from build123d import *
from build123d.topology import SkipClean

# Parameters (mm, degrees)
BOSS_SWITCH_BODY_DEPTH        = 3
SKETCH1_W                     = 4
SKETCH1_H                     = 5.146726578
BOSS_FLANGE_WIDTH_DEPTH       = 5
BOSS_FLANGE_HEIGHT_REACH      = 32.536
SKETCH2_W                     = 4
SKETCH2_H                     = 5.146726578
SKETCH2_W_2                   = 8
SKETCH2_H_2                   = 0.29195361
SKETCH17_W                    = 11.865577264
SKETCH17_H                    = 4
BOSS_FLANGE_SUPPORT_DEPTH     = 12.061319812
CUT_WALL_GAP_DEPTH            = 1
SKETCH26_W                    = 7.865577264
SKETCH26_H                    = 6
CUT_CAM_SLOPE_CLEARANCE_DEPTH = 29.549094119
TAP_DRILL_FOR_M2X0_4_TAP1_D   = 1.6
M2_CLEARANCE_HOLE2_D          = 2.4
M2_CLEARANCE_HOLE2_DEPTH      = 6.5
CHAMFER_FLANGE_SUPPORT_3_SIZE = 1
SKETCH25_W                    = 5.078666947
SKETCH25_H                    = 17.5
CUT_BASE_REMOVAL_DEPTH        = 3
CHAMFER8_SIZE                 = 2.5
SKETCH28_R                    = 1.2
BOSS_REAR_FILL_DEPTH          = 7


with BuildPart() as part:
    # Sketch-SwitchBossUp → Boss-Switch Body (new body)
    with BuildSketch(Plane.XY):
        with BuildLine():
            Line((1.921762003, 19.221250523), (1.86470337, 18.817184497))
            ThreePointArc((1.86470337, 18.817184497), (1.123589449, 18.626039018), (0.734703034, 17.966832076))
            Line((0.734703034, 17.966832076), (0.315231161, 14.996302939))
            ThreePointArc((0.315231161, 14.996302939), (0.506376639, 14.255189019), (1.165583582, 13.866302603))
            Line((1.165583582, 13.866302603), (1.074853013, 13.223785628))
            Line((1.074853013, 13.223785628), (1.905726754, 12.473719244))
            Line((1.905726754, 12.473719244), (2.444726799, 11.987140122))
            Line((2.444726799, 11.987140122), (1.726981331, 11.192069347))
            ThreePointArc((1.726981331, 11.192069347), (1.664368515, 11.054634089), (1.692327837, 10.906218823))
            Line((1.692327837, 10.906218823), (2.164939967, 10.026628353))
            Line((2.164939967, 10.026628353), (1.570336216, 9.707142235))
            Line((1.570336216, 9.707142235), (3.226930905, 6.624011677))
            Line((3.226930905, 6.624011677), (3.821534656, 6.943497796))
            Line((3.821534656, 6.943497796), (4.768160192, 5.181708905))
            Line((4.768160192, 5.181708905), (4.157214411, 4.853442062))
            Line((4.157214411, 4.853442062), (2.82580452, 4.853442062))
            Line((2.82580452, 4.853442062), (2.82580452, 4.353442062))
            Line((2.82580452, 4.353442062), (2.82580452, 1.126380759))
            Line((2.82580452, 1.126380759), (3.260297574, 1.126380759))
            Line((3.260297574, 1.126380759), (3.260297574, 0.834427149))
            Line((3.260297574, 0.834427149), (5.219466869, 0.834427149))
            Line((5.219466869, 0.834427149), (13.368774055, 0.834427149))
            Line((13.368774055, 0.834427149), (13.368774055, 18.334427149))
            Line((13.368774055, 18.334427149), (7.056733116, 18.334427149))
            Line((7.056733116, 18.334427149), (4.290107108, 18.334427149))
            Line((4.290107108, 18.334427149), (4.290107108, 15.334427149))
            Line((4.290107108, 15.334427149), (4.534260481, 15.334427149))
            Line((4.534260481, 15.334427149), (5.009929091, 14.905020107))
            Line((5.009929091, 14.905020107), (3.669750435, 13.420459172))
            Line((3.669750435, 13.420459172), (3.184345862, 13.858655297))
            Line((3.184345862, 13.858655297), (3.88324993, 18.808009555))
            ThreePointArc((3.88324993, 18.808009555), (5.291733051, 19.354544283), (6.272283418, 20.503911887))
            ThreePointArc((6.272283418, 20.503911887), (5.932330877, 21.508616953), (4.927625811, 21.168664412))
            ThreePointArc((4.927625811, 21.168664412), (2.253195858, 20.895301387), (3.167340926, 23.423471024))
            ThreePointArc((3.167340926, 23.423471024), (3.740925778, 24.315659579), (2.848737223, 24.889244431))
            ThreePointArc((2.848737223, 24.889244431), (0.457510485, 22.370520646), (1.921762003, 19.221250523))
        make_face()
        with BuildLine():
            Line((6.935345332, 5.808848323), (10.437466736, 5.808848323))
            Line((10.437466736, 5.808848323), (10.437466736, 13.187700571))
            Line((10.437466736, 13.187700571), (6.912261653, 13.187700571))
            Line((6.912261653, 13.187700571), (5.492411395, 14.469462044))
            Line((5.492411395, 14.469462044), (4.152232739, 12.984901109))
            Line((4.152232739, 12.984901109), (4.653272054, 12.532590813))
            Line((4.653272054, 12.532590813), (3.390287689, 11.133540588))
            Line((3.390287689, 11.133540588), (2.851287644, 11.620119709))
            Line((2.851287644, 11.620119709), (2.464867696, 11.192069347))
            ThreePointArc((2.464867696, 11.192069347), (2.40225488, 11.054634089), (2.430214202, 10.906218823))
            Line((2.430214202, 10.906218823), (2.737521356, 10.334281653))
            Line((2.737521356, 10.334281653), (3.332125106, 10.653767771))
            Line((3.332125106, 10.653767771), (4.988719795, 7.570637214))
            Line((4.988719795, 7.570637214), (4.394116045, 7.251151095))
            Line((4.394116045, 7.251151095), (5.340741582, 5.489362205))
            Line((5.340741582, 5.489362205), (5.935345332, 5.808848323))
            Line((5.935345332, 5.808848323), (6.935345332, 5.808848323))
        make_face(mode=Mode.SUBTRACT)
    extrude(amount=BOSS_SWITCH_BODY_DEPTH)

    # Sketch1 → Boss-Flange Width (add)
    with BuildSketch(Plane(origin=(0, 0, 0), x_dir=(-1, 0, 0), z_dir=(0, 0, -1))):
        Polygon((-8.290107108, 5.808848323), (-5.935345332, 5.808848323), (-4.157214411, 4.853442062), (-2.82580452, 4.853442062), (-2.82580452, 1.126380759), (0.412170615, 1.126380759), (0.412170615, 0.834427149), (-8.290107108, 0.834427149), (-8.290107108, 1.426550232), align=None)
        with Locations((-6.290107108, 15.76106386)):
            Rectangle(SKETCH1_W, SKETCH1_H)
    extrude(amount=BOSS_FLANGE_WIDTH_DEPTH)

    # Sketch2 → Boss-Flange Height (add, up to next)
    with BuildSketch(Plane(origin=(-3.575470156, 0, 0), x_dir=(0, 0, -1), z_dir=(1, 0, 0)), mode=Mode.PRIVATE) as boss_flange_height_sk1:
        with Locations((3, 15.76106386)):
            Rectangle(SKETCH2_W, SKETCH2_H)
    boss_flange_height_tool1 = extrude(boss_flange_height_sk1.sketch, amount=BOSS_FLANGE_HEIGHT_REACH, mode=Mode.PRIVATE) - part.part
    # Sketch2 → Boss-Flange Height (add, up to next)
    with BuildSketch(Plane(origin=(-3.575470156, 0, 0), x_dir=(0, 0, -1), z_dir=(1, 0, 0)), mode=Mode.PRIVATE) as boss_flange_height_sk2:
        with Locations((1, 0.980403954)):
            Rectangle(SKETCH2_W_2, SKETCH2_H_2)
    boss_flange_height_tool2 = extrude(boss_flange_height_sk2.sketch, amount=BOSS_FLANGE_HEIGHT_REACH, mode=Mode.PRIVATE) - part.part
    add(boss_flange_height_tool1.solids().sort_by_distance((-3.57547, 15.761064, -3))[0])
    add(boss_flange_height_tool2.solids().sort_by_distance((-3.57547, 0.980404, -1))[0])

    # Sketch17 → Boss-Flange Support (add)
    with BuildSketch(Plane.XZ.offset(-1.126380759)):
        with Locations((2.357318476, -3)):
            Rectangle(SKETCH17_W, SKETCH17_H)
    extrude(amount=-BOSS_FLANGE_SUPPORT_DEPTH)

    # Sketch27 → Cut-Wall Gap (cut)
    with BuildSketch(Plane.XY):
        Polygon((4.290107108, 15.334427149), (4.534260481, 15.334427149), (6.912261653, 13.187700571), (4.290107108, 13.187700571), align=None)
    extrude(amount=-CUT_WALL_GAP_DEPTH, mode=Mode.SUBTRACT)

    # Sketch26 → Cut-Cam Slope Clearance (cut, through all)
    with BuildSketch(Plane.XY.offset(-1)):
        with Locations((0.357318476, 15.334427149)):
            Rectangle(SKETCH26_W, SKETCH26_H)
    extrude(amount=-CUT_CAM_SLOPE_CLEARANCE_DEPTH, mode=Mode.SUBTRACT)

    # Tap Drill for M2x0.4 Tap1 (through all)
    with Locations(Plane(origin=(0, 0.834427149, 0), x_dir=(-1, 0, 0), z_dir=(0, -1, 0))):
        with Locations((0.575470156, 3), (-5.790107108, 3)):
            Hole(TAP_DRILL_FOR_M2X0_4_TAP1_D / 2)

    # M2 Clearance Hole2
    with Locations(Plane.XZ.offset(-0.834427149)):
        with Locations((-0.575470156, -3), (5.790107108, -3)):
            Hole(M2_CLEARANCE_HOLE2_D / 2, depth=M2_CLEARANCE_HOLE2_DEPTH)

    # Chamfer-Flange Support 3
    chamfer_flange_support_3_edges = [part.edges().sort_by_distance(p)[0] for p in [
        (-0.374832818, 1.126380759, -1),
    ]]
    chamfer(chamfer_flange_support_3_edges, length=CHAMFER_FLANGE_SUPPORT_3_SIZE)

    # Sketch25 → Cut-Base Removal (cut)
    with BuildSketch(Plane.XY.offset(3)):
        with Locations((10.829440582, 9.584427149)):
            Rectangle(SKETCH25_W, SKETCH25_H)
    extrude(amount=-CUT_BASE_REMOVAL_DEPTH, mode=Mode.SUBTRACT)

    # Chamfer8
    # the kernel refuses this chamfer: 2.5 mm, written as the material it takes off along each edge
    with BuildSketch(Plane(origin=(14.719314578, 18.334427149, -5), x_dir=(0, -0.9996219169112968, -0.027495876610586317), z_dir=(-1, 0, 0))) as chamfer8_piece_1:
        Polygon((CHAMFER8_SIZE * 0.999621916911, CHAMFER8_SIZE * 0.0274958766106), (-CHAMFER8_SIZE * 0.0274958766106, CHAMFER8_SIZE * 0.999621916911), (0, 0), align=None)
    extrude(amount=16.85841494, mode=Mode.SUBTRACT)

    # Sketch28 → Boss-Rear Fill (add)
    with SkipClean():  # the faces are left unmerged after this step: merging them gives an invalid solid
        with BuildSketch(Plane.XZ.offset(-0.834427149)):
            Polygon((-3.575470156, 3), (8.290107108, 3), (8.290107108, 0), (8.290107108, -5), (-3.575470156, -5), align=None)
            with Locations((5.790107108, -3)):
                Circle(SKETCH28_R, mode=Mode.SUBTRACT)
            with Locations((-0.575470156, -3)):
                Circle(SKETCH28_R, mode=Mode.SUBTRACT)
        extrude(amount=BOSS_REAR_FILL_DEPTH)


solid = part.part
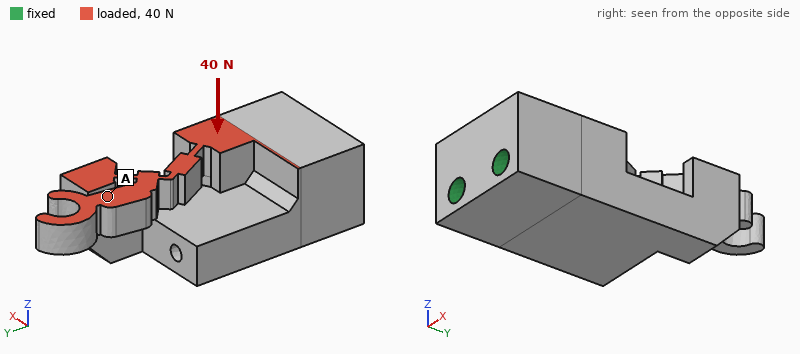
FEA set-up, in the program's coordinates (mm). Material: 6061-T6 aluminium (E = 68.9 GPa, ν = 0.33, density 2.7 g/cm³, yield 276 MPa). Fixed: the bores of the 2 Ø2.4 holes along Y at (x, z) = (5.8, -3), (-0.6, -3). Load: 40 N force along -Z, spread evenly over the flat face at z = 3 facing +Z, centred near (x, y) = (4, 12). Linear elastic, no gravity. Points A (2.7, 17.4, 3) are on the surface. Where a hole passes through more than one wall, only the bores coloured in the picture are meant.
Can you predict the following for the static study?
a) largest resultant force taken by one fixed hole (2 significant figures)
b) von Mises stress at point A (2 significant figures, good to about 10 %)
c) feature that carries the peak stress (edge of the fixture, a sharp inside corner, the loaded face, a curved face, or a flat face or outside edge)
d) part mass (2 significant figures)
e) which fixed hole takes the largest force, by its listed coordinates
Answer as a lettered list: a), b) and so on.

a) 30 N
b) 7.9 MPa
c) a curved face
d) 3.9 g
e) (5.8, -3)
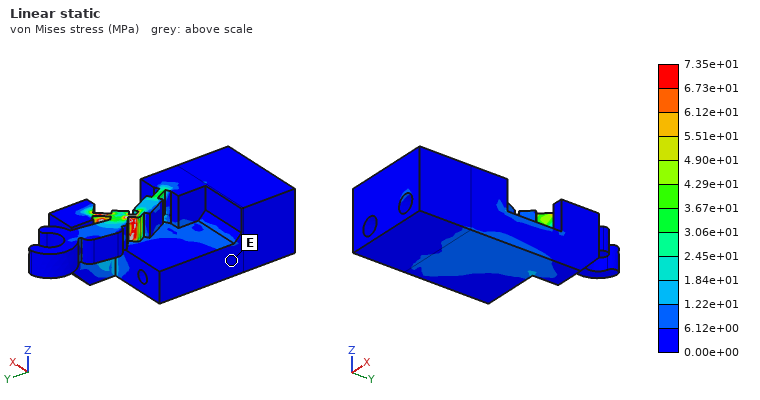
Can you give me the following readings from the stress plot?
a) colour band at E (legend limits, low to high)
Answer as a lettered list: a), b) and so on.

a) 0.00e+00 to 6.12e+00 MPa
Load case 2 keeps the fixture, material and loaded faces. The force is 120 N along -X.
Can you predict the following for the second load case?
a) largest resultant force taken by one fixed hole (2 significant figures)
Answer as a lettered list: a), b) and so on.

a) 220 N
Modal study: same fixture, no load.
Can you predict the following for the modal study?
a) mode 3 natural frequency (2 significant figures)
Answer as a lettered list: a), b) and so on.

a) 13 kHz
